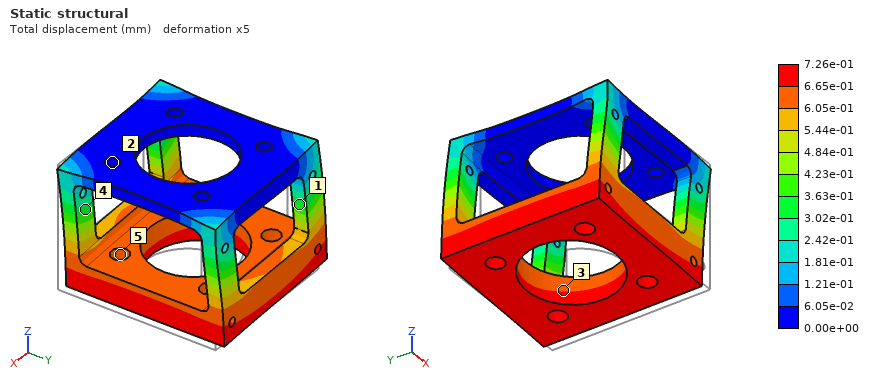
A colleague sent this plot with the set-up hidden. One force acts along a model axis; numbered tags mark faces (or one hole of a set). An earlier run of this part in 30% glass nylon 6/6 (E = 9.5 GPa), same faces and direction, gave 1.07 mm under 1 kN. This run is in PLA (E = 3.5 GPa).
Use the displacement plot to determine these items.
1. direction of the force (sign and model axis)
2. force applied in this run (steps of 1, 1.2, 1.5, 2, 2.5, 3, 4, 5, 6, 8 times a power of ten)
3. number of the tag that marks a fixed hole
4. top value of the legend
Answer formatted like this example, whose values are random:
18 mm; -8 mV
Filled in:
-X; 250 N; 2; 7.26e-01 mm
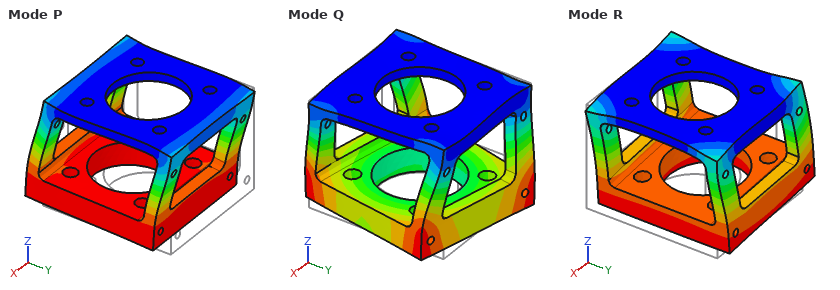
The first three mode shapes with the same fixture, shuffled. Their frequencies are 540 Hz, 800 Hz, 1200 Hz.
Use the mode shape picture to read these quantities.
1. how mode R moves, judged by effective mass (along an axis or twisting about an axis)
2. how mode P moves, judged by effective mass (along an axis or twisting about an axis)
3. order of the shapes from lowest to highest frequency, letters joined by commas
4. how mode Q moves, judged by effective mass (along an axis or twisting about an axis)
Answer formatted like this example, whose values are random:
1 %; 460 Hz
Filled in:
along X; along Y; P, R, Q; twisting about Z
